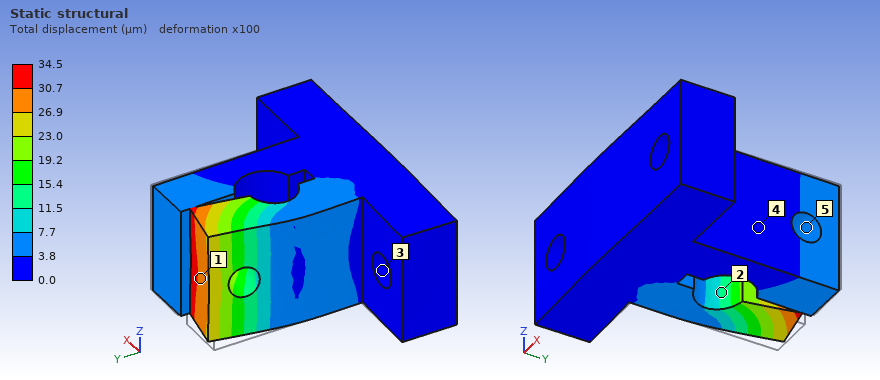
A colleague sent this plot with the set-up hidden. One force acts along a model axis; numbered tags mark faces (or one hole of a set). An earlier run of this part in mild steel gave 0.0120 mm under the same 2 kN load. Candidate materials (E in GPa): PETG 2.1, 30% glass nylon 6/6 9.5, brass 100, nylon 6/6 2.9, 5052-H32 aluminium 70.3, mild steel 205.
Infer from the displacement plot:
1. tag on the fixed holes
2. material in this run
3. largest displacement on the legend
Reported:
3
5052-H32 aluminium
34.5 µm
